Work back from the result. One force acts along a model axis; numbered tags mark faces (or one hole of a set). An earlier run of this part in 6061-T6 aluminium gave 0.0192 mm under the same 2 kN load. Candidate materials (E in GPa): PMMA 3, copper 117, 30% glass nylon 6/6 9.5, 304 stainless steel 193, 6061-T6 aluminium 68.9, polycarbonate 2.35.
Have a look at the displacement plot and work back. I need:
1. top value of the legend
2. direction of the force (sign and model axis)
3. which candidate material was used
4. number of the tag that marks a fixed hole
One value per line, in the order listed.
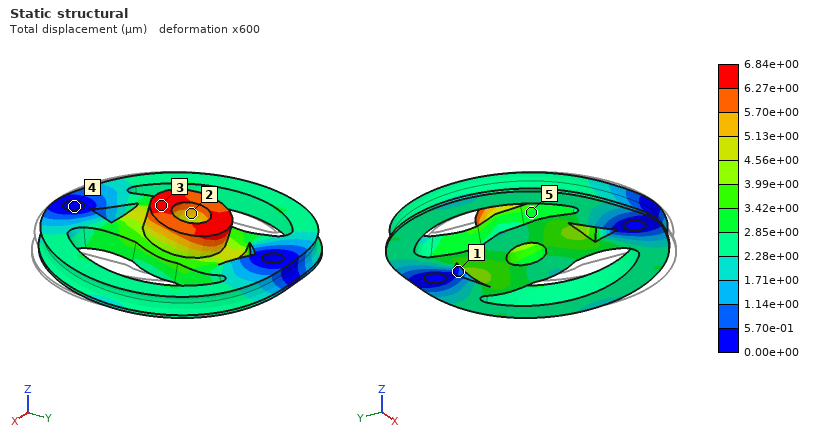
6.84e+00 µm
+Y
304 stainless steel
4
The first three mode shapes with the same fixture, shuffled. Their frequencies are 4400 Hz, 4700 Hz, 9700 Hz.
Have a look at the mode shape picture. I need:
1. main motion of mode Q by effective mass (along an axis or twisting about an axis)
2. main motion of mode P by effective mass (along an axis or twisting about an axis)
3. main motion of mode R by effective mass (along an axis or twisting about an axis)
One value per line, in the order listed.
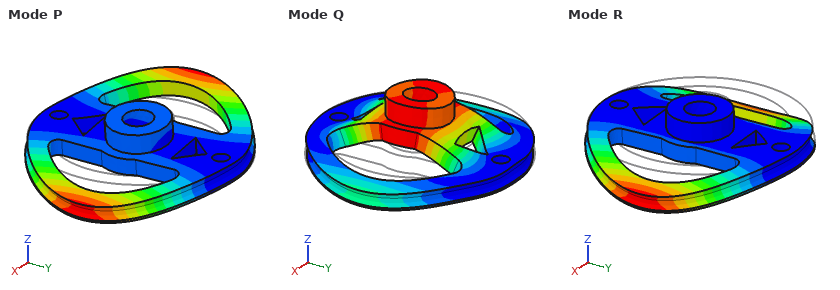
along Z
twisting about Y
along Z
